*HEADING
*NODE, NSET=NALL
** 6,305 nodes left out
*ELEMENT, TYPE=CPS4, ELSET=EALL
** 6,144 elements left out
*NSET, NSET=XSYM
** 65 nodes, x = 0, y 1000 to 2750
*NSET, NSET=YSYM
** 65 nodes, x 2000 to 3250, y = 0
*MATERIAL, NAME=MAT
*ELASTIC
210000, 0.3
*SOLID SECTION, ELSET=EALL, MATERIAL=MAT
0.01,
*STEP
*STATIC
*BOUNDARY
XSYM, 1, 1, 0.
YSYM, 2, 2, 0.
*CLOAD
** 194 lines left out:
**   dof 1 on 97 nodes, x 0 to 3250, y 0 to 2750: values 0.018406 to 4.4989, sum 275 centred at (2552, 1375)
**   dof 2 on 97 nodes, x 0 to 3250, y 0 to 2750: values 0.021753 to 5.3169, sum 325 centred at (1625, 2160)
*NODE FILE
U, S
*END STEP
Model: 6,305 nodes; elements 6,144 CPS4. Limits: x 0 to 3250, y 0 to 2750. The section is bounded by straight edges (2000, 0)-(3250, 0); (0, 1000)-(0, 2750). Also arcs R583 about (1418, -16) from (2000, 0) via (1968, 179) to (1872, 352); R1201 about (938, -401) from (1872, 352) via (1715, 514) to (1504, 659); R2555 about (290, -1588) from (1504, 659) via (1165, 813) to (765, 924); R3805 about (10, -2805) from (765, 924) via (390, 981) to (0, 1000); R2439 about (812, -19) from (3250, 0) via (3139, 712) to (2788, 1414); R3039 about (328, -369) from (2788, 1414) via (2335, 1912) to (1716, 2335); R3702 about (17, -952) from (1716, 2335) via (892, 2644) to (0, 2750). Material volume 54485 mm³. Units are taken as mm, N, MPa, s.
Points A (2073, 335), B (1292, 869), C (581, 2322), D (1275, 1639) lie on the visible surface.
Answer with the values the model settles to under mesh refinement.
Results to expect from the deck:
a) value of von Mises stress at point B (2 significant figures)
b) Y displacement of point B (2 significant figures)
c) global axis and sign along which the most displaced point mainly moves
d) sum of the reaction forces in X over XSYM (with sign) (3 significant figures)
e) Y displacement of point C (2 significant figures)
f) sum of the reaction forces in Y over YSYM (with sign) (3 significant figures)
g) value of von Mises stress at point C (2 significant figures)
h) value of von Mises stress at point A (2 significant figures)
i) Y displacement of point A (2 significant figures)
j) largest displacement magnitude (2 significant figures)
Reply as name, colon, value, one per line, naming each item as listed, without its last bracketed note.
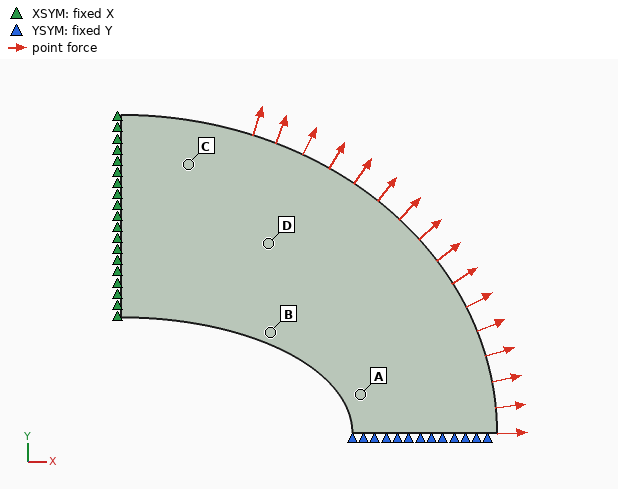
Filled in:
value of von Mises stress at point B: 12 MPa
Y displacement of point B: 0.39 mm
global axis and sign along which the most displaced point mainly moves: +Y
sum of the reaction forces in X over XSYM (with sign): -275 N
Y displacement of point C: 0.52 mm
sum of the reaction forces in Y over YSYM (with sign): -325 N
value of von Mises stress at point C: 23 MPa
value of von Mises stress at point A: 45 MPa
Y displacement of point A: 0.090 mm
largest displacement magnitude: 0.55 mm
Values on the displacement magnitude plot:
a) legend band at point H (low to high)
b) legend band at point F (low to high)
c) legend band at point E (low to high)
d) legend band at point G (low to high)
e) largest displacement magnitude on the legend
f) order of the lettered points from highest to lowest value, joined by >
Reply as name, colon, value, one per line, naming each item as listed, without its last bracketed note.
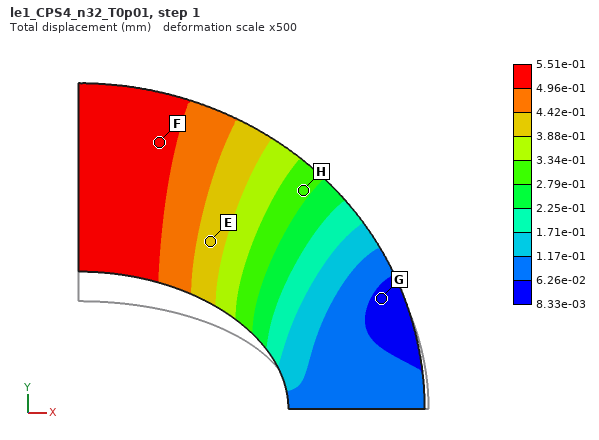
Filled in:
legend band at point H: 2.79e-01 to 3.34e-01 mm
legend band at point F: 4.96e-01 to 5.51e-01 mm
legend band at point E: 3.88e-01 to 4.42e-01 mm
legend band at point G: 8.33e-03 to 6.26e-02 mm
largest displacement magnitude on the legend: 5.51e-01 mm
order of the lettered points from highest to lowest value, joined by >: F > E > H > G
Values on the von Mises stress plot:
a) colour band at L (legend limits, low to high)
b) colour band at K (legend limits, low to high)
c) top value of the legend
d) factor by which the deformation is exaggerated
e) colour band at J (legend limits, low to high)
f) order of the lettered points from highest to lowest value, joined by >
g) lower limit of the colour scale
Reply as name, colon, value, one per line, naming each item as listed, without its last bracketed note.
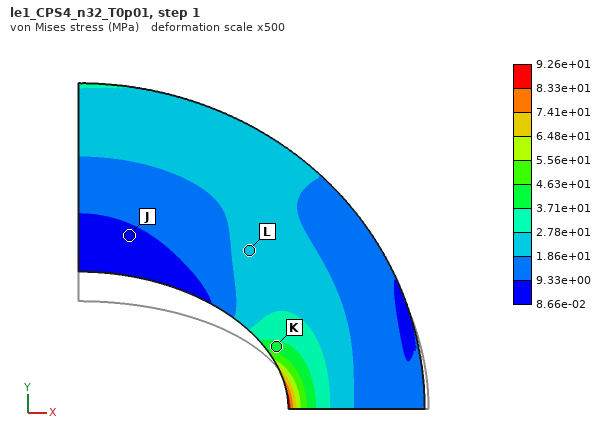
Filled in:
colour band at L: 1.86e+01 to 2.78e+01 MPa
colour band at K: 3.71e+01 to 4.63e+01 MPa
top value of the legend: 9.26e+01 MPa
factor by which the deformation is exaggerated: 500
colour band at J: 8.66e-02 to 9.33e+00 MPa
order of the lettered points from highest to lowest value, joined by >: K > L > J
lower limit of the colour scale: 8.66e-02 MPa
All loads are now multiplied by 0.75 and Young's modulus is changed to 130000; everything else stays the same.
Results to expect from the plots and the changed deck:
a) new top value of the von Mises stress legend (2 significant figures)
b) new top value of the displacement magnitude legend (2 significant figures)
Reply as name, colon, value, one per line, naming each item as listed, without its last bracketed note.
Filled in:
new top value of the von Mises stress legend: 69 MPa
new top value of the displacement magnitude legend: 0.67 mm
